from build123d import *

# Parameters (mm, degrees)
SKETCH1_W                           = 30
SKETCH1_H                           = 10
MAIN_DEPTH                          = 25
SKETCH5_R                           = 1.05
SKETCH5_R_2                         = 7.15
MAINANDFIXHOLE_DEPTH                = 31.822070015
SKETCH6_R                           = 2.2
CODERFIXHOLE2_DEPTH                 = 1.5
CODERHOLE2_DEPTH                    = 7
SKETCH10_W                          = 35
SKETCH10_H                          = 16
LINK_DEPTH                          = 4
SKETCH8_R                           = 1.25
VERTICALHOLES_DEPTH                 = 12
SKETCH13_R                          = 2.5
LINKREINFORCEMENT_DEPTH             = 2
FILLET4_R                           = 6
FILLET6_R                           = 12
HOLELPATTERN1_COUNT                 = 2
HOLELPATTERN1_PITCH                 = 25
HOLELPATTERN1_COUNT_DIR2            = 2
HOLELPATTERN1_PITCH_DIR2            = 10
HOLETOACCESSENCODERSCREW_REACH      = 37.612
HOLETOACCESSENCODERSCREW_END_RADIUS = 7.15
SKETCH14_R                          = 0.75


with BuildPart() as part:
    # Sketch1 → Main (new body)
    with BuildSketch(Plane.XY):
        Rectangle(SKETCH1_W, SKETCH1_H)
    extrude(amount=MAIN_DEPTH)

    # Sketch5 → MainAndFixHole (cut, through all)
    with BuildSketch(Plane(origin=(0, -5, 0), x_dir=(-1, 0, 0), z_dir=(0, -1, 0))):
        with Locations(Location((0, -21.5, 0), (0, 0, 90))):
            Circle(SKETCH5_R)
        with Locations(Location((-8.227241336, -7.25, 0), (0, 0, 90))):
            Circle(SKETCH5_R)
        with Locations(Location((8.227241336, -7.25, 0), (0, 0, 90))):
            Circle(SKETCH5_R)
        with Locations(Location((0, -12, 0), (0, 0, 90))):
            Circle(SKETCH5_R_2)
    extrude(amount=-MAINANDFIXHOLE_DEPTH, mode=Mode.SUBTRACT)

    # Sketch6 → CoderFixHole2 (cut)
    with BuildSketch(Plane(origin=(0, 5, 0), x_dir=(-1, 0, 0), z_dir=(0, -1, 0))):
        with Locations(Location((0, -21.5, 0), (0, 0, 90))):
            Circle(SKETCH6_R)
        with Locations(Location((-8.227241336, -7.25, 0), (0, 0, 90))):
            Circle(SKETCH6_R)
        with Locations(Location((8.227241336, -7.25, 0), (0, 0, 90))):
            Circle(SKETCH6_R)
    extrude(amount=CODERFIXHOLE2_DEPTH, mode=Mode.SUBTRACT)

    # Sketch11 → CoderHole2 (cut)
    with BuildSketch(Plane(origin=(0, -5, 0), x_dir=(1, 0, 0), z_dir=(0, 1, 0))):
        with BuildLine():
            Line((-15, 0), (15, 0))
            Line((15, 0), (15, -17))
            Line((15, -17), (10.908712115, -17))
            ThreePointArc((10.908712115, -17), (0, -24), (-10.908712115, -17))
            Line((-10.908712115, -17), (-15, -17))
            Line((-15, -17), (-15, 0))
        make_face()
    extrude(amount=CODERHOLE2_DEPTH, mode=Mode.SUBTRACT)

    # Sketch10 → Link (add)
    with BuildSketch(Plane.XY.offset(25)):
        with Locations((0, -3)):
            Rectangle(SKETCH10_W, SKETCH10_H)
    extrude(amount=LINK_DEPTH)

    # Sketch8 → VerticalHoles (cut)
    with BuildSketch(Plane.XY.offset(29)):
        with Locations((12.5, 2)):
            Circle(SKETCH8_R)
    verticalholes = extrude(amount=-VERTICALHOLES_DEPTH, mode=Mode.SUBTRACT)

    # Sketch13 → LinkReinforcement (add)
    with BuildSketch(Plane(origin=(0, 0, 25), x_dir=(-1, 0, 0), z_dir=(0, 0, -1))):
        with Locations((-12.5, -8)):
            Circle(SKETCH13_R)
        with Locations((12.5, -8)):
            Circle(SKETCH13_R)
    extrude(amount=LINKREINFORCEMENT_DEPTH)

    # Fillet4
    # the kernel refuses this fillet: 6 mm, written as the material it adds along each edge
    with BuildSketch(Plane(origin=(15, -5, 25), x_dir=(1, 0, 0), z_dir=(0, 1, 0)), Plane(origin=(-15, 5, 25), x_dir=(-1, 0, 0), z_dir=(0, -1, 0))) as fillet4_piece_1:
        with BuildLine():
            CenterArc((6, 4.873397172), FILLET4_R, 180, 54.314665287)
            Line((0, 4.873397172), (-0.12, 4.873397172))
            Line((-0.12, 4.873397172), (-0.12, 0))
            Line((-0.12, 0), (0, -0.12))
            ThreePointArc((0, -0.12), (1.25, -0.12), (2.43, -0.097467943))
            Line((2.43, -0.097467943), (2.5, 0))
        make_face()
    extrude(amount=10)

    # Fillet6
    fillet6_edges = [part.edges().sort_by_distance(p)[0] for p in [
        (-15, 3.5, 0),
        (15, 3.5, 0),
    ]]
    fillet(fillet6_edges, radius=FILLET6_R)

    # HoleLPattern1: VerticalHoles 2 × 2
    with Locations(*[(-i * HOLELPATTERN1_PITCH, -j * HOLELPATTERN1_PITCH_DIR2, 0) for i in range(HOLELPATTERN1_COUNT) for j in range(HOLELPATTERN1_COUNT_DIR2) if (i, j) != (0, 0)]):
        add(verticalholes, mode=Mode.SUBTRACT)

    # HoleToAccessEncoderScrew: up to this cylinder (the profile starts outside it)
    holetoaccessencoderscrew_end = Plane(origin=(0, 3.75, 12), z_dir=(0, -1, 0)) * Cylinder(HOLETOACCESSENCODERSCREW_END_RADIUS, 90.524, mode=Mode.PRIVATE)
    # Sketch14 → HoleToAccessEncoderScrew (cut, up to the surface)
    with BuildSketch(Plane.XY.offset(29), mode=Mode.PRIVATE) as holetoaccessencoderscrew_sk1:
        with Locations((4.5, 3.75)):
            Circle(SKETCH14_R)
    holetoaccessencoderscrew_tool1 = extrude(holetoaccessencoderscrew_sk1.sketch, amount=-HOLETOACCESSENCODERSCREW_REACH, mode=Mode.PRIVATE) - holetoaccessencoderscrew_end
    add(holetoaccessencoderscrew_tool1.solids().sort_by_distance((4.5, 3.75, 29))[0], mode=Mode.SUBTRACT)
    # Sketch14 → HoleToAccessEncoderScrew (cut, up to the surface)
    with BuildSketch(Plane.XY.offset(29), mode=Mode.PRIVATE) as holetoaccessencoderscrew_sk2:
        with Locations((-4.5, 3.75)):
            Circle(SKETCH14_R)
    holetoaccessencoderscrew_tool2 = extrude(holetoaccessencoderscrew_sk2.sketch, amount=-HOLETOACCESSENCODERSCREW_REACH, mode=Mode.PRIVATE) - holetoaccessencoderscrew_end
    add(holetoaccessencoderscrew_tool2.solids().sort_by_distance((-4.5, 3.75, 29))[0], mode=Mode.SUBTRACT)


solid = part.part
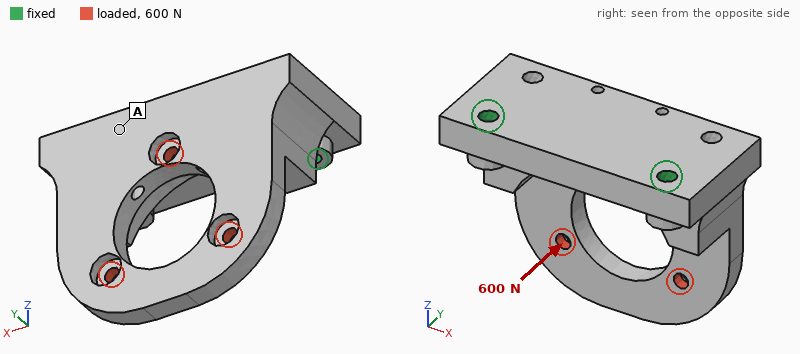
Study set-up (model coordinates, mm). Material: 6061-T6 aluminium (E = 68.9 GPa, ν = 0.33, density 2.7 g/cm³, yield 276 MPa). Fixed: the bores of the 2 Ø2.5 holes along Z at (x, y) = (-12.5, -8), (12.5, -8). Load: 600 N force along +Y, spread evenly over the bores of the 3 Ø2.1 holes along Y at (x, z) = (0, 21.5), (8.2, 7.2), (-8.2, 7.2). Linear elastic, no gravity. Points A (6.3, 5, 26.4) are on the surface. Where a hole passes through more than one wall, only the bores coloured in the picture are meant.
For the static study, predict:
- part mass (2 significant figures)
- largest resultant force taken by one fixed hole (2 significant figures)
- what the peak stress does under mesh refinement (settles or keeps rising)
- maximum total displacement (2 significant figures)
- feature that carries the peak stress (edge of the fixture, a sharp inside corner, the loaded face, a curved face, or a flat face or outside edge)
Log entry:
12 g
330 N
keeps rising
0.35 mm
a sharp inside corner
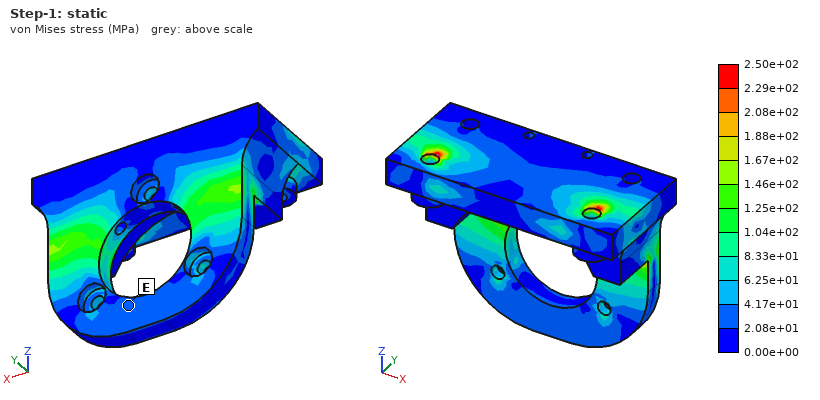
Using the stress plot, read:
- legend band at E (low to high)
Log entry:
2.08e+01 to 4.17e+01 MPa
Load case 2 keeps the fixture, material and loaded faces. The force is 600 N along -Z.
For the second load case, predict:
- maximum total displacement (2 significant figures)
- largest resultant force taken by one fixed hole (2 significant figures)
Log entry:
63 µm
300 N
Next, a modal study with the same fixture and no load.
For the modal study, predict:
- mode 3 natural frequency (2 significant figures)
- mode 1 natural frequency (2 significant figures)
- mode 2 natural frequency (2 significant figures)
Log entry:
10 kHz
4300 Hz
9600 Hz
